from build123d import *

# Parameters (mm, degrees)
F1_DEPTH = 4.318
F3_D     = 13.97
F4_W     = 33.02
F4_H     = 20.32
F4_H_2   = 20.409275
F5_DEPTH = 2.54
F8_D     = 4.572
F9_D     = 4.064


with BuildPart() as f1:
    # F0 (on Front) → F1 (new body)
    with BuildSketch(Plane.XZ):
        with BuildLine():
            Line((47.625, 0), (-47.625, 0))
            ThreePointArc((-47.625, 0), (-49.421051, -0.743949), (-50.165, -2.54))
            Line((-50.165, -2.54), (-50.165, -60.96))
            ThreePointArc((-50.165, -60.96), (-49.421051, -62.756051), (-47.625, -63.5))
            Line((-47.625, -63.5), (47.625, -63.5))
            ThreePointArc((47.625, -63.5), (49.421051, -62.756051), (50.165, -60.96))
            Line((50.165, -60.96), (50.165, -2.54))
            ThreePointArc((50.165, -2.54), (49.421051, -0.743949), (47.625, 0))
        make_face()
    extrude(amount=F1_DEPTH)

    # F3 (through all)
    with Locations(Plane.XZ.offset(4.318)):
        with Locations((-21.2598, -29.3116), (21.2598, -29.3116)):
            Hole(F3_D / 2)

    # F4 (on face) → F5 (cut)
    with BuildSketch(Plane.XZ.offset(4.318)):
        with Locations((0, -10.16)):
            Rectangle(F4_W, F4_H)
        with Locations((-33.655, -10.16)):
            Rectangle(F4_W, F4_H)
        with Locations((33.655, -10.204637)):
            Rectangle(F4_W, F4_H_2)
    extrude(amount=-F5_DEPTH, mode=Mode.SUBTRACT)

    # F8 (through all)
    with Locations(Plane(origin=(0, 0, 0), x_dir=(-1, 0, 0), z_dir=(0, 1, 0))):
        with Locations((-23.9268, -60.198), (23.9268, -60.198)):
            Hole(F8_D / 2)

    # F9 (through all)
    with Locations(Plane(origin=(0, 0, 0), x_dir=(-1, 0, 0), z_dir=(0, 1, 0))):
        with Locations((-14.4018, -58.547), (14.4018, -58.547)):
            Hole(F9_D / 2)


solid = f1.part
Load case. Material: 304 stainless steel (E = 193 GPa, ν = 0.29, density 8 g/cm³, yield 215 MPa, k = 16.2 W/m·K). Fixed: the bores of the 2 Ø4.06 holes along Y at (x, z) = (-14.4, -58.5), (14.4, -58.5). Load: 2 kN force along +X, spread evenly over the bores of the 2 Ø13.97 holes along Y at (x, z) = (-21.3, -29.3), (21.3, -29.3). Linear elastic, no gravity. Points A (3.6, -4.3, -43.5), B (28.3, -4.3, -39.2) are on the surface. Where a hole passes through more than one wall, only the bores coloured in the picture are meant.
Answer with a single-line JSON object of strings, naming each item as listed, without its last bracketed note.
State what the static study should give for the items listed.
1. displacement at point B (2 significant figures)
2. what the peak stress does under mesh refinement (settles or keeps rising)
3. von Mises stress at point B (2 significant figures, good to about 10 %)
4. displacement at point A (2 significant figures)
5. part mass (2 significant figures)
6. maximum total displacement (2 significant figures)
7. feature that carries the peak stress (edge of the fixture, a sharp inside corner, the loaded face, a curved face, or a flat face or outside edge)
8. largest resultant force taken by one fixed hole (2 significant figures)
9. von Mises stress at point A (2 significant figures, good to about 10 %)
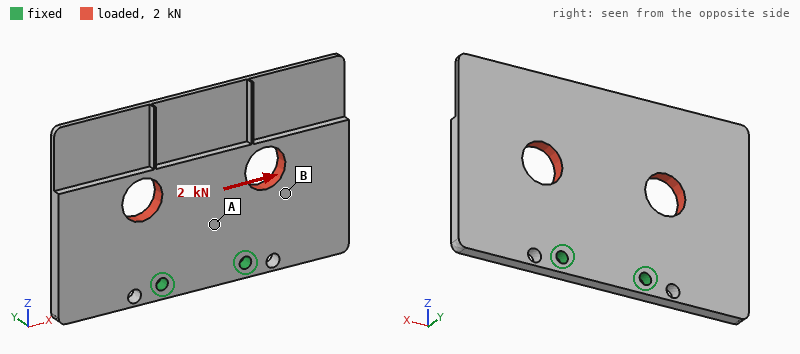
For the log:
{"displacement at point B": "8.2 µm", "what the peak stress does under mesh refinement": "keeps rising", "von Mises stress at point B": "7.8 MPa", "displacement at point A": "4.0 µm", "part mass": "170 g", "maximum total displacement": "19 µm", "feature that carries the peak stress": "edge of the fixture", "largest resultant force taken by one fixed hole": "2.1 kN", "von Mises stress at point A": "23 MPa"}
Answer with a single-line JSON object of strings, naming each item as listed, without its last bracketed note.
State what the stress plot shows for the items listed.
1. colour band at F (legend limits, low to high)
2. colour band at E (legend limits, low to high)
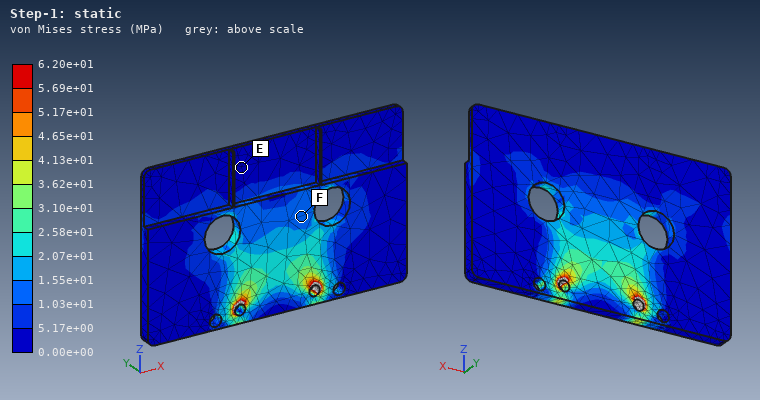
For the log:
{"colour band at F": "1.03e+01 to 1.55e+01 MPa", "colour band at E": "0.00e+00 to 5.17e+00 MPa"}
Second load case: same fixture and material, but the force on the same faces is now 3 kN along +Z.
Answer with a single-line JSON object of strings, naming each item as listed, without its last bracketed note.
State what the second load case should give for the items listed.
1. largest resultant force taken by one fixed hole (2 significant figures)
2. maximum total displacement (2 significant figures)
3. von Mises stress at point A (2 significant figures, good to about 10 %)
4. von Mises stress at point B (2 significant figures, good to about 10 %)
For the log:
{"largest resultant force taken by one fixed hole": "1.5 kN", "maximum total displacement": "5.1 µm", "von Mises stress at point A": "9.5 MPa", "von Mises stress at point B": "13 MPa"}
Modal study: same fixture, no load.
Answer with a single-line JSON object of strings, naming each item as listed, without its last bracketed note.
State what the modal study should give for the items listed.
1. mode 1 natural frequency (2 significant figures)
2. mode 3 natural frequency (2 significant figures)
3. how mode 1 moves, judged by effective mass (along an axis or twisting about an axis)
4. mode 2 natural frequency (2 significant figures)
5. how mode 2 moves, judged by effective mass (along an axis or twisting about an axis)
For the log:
{"mode 1 natural frequency": "1000 Hz", "mode 3 natural frequency": "2000 Hz", "how mode 1 moves, judged by effective mass": "along Y", "mode 2 natural frequency": "1200 Hz", "how mode 2 moves, judged by effective mass": "twisting about Z"}
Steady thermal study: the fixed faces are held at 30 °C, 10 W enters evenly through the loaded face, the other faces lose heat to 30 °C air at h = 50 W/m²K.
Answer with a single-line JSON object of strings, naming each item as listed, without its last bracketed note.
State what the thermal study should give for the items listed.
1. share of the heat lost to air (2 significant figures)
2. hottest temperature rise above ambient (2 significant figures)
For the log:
{"share of the heat lost to air": "77 %", "hottest temperature rise above ambient": "29 K"}
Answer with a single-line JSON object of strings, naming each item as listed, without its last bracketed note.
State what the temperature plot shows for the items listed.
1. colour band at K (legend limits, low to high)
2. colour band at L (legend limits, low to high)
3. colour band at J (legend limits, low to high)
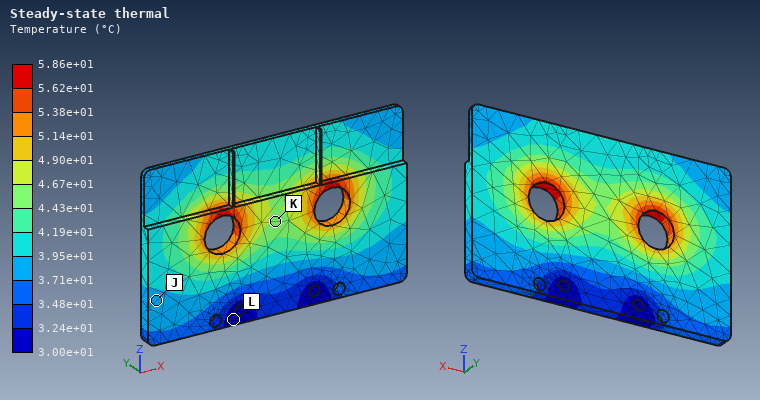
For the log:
{"colour band at K": "4.43e+01 to 4.67e+01 °C", "colour band at L": "3.00e+01 to 3.24e+01 °C", "colour band at J": "3.71e+01 to 3.95e+01 °C"}
